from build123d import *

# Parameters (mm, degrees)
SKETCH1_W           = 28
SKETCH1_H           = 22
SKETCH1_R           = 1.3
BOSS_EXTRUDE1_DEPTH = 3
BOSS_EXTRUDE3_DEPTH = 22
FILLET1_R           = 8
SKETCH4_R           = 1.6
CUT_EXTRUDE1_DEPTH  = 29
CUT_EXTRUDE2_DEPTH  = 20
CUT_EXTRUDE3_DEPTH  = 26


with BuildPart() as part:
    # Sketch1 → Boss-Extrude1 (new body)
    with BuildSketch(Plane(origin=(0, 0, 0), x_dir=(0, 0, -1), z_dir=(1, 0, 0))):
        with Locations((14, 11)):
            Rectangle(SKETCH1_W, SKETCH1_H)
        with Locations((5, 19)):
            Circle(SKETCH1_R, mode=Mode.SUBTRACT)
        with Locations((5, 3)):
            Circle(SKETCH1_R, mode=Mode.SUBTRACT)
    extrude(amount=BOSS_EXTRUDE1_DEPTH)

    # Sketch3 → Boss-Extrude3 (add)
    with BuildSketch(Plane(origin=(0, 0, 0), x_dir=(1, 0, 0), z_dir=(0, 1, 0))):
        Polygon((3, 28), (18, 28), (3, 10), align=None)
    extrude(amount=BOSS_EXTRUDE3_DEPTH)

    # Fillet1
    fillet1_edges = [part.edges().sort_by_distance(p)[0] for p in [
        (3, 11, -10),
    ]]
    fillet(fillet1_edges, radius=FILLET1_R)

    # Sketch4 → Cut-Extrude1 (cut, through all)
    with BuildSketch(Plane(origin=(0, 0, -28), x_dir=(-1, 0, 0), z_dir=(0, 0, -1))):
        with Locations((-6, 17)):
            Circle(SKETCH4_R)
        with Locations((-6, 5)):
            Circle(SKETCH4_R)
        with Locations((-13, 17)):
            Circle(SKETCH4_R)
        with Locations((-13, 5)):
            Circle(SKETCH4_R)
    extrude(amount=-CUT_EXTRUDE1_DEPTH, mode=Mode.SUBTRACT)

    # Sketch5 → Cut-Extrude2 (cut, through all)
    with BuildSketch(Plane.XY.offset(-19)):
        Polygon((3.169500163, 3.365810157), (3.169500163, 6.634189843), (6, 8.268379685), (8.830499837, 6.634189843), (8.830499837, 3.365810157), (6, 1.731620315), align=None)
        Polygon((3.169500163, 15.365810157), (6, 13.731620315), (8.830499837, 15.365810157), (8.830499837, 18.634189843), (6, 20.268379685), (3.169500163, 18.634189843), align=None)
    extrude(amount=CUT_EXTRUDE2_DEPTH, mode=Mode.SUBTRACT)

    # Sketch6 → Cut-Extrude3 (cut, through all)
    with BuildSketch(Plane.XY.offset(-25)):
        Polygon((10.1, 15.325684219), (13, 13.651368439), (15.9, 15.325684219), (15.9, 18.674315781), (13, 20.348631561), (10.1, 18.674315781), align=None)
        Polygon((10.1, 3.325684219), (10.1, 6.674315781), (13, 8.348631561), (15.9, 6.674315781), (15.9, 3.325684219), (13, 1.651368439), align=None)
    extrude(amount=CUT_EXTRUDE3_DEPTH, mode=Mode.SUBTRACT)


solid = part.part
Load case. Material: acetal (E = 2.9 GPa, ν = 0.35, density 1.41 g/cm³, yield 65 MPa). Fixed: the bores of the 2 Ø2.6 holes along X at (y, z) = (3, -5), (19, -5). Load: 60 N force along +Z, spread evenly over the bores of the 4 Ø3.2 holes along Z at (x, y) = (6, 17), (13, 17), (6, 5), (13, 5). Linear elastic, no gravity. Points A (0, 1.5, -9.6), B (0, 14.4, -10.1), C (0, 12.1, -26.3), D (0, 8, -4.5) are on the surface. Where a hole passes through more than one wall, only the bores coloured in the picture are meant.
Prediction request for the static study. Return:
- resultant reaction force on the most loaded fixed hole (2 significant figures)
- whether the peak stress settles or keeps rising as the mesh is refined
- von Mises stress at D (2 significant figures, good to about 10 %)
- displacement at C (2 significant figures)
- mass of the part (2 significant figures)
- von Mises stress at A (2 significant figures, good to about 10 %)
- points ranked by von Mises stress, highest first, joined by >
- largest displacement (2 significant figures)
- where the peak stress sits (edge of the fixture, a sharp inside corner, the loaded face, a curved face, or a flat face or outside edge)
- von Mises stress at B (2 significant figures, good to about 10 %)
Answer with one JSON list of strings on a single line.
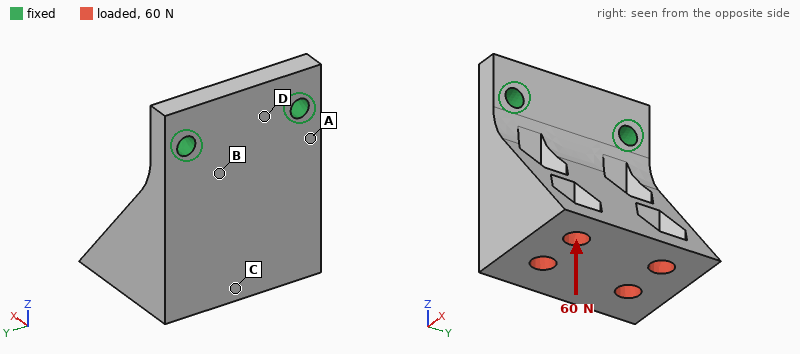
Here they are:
["30 N", "keeps rising", "3.5 MPa", "0.31 mm", "5.8 g", "8.9 MPa", "A > B > D > C", "0.45 mm", "edge of the fixture", "6.3 MPa"]
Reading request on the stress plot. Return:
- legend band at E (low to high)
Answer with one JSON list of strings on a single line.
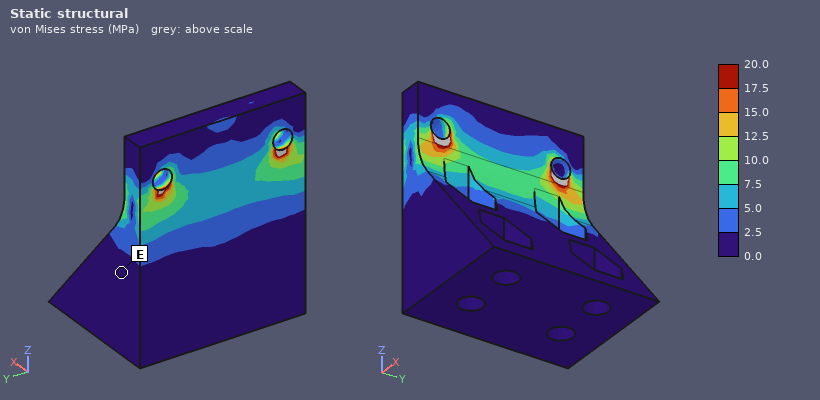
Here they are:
["0.0 to 2.5 MPa"]
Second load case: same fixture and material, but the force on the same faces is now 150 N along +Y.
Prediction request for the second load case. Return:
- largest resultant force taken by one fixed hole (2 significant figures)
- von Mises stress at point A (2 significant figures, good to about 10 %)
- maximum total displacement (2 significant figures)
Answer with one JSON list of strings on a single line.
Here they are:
["190 N", "7.2 MPa", "0.24 mm"]
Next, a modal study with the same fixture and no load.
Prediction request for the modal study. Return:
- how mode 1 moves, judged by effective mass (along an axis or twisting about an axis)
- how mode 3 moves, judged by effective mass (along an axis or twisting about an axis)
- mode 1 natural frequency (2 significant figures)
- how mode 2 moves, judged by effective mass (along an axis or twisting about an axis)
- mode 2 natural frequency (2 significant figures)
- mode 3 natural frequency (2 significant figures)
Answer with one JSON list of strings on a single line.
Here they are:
["along X", "along Y", "690 Hz", "along Y", "2400 Hz", "4000 Hz"]
